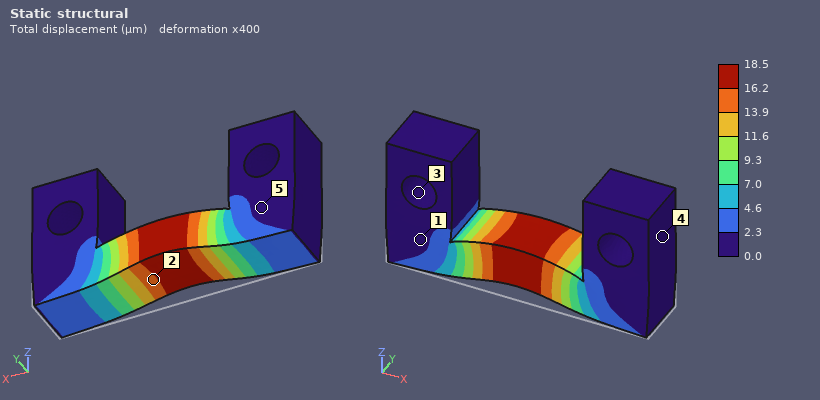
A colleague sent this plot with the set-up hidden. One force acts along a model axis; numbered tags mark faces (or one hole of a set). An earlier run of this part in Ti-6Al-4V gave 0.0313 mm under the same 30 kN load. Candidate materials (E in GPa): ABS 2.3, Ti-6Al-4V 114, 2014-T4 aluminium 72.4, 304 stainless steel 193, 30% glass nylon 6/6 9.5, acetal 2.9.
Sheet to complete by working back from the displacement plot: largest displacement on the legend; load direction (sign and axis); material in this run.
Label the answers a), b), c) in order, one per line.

a) 18.5 µm
b) +Z
c) 304 stainless steel
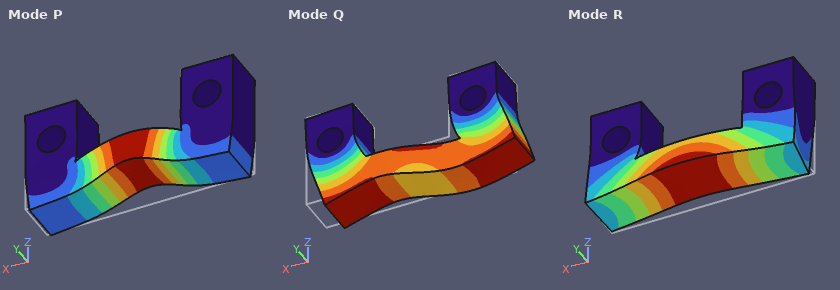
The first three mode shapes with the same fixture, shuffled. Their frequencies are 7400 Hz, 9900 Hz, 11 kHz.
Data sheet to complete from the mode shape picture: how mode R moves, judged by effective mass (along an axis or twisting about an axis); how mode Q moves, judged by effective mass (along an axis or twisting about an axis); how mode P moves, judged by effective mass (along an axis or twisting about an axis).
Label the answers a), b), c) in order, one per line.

a) along Y
b) along X
c) along Z
